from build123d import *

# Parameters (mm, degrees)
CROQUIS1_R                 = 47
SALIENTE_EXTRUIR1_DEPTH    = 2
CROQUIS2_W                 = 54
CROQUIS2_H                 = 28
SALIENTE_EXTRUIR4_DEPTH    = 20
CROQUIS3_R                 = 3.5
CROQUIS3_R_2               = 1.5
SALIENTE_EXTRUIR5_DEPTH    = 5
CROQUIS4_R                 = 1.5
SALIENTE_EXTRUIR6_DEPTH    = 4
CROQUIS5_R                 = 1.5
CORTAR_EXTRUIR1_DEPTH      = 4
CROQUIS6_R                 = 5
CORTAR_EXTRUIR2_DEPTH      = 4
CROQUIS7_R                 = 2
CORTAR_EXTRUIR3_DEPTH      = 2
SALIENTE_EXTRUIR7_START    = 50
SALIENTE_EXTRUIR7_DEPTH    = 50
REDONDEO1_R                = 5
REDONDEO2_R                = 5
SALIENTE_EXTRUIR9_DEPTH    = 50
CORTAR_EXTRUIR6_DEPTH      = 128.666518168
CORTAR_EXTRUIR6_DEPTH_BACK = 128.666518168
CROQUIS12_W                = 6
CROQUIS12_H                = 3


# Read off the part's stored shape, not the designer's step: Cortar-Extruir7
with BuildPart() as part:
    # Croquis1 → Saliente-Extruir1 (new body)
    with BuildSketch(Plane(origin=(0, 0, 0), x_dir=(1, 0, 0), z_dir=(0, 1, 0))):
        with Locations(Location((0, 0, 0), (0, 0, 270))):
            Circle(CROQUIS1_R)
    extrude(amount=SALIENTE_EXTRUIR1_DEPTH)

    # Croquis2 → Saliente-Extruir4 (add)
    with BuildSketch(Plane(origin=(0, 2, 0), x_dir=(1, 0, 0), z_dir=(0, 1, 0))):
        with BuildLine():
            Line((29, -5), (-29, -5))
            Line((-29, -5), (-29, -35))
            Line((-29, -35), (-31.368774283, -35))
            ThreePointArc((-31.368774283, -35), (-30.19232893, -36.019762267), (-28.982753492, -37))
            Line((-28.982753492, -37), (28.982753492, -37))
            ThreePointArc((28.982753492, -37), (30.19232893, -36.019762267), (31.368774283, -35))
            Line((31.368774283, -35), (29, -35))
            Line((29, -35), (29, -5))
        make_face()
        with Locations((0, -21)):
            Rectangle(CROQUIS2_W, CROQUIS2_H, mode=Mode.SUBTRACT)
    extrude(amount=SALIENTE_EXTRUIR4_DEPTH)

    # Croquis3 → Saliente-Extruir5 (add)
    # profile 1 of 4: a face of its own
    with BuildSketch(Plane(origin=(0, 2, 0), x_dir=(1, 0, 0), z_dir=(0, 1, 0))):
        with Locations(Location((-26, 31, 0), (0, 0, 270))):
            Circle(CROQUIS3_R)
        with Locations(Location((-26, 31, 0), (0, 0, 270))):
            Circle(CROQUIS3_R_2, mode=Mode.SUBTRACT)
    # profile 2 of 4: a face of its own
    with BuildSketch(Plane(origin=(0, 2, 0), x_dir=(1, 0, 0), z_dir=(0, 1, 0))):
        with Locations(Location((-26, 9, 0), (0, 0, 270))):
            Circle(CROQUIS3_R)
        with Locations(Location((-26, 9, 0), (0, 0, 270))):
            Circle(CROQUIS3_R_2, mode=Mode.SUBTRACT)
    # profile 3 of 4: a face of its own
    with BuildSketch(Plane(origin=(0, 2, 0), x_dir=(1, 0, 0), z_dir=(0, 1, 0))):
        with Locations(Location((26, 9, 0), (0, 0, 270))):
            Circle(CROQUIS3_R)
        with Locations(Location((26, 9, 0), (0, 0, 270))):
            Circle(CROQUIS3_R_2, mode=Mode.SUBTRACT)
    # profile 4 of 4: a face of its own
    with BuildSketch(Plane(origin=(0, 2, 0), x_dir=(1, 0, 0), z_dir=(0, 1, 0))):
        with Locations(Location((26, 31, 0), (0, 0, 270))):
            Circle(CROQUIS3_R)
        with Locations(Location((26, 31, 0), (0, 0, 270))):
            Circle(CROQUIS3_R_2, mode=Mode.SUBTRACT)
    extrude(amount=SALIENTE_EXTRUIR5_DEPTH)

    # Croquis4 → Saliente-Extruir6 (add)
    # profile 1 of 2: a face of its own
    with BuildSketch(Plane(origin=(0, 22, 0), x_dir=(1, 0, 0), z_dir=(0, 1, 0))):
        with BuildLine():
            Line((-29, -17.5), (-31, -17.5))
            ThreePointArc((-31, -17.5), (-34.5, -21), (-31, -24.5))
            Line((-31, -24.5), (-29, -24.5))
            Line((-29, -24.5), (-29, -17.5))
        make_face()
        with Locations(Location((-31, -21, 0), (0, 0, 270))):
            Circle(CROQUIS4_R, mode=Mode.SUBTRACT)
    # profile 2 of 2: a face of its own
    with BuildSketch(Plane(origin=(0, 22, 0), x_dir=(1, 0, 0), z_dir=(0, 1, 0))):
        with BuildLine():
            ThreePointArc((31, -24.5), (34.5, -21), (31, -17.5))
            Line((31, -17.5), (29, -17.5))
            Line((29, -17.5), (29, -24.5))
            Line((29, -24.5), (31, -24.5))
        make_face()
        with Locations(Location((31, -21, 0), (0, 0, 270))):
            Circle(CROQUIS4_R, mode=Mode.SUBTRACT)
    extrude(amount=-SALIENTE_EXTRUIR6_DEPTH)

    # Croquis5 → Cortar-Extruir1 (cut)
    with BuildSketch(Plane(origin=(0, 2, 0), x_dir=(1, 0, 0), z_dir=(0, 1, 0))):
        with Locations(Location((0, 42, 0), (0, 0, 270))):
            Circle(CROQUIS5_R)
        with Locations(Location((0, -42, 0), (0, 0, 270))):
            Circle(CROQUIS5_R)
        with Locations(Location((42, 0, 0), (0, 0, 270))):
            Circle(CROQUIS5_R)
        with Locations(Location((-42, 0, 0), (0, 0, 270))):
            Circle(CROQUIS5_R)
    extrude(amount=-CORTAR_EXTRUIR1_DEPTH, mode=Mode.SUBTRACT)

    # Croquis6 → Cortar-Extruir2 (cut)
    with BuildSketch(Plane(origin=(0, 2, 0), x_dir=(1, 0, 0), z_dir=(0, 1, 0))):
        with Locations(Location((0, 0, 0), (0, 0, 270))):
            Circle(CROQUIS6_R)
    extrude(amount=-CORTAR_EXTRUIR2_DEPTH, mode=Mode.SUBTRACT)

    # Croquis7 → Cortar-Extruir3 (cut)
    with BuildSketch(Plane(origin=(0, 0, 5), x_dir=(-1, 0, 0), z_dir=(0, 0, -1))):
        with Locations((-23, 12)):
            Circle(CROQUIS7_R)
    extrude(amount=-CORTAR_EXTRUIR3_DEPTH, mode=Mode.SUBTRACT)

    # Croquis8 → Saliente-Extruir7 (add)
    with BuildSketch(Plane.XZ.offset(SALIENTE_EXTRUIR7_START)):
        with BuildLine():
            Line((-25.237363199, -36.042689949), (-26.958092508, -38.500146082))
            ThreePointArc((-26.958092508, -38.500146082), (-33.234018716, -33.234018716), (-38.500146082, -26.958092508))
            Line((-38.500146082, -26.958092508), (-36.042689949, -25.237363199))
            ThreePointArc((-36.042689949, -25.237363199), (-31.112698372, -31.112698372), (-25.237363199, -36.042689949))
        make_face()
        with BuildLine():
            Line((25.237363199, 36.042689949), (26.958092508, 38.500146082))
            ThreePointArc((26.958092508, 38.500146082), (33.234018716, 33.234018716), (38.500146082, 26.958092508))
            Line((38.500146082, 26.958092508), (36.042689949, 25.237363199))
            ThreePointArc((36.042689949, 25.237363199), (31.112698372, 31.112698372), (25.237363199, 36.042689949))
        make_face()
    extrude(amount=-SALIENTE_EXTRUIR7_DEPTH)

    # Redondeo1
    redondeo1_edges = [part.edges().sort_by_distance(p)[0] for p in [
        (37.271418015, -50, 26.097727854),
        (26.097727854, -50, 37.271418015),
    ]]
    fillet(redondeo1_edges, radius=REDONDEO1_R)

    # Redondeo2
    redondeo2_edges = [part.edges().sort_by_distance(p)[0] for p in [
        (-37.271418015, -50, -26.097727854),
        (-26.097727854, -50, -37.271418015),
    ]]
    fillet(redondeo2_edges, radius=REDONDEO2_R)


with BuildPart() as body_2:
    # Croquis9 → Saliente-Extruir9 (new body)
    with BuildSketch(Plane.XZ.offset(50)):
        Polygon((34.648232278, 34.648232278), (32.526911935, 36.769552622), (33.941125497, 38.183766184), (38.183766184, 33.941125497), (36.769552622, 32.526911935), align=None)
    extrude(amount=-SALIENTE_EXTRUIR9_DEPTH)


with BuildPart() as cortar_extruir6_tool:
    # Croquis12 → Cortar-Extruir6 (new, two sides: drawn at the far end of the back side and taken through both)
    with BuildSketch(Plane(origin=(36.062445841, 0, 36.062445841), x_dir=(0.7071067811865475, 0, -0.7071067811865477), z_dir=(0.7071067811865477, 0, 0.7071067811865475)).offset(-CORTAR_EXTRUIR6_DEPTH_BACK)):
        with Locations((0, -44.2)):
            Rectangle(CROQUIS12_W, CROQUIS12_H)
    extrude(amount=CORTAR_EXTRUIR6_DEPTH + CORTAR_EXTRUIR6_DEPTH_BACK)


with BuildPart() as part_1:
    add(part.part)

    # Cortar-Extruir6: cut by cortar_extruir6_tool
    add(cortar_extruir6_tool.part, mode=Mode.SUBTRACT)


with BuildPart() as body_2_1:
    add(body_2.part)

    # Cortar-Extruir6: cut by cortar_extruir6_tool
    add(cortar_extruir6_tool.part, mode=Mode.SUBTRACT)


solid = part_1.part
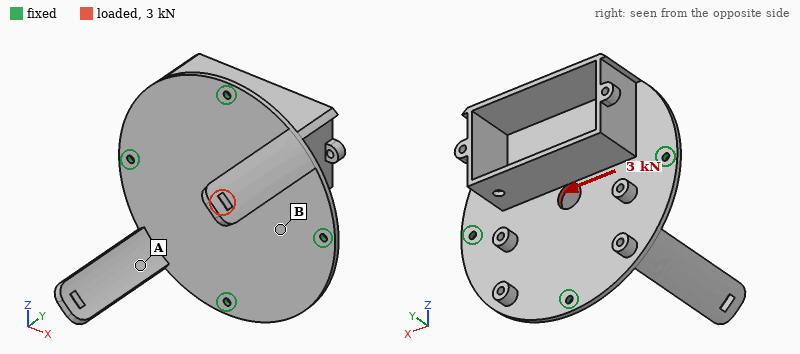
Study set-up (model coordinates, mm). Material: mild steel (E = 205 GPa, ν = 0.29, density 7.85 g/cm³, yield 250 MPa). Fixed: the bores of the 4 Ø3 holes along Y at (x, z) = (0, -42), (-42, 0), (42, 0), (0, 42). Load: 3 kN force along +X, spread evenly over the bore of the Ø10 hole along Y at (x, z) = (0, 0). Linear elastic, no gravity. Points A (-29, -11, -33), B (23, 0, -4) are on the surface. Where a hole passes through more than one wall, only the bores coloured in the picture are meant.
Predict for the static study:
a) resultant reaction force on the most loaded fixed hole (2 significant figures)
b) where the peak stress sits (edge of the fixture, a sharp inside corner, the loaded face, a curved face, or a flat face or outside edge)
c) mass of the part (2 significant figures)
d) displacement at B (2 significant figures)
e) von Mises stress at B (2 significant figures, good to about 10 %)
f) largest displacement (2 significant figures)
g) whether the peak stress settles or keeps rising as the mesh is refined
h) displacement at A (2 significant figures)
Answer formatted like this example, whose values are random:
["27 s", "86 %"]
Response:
["940 N", "edge of the fixture", "200 g", "3.1 µm", "27 MPa", "6.1 µm", "keeps rising", "2.4 µm"]
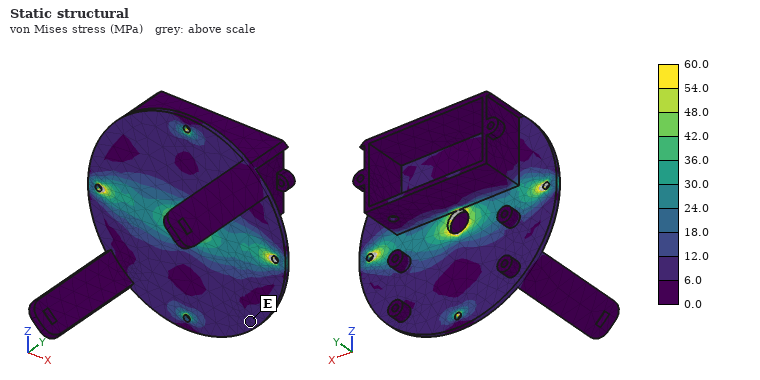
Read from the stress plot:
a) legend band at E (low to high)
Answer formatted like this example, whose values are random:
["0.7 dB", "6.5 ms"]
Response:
["6.0 to 12.0 MPa"]
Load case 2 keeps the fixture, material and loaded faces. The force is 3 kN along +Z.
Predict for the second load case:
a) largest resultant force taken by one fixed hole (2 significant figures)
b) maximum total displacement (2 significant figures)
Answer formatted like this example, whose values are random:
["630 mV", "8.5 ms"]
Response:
["940 N", "6.9 µm"]
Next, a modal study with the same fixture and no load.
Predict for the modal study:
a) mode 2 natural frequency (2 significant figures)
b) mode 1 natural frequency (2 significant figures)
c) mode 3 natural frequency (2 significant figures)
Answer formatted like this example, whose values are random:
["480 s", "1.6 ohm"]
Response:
["800 Hz", "570 Hz", "1100 Hz"]
